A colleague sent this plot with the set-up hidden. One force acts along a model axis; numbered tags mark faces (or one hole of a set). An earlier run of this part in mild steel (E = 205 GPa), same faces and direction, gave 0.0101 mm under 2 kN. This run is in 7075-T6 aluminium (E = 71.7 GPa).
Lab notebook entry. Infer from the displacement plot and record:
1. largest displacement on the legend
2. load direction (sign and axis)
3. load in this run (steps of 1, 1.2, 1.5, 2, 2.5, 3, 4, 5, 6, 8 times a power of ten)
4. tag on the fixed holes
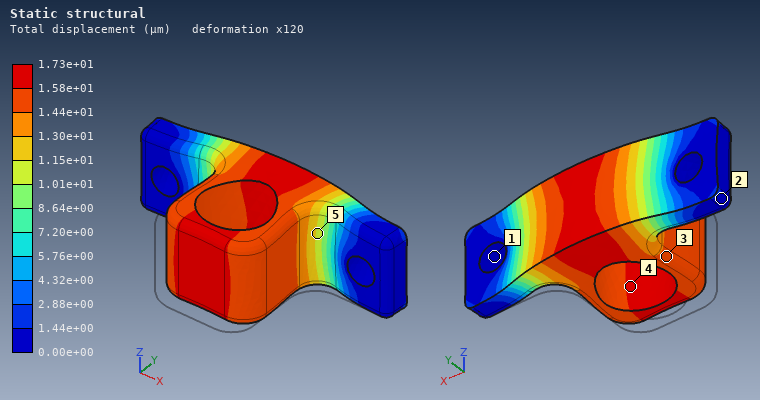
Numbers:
1.73e+01 µm
+Y
1.2 kN
1
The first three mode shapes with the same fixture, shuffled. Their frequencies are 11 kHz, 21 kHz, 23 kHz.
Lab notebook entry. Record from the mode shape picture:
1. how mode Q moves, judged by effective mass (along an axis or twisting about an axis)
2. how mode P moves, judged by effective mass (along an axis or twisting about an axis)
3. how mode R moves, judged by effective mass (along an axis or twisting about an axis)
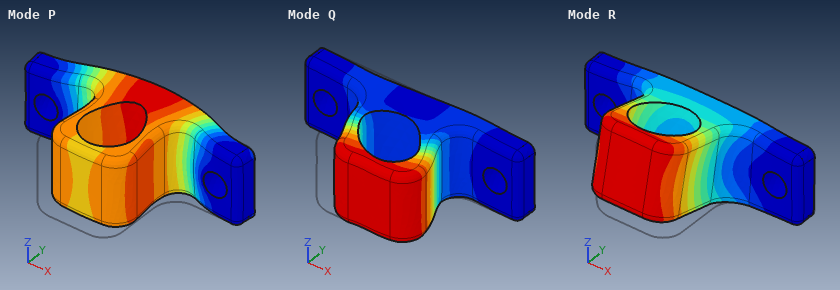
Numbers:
along X
along Y
along Z
